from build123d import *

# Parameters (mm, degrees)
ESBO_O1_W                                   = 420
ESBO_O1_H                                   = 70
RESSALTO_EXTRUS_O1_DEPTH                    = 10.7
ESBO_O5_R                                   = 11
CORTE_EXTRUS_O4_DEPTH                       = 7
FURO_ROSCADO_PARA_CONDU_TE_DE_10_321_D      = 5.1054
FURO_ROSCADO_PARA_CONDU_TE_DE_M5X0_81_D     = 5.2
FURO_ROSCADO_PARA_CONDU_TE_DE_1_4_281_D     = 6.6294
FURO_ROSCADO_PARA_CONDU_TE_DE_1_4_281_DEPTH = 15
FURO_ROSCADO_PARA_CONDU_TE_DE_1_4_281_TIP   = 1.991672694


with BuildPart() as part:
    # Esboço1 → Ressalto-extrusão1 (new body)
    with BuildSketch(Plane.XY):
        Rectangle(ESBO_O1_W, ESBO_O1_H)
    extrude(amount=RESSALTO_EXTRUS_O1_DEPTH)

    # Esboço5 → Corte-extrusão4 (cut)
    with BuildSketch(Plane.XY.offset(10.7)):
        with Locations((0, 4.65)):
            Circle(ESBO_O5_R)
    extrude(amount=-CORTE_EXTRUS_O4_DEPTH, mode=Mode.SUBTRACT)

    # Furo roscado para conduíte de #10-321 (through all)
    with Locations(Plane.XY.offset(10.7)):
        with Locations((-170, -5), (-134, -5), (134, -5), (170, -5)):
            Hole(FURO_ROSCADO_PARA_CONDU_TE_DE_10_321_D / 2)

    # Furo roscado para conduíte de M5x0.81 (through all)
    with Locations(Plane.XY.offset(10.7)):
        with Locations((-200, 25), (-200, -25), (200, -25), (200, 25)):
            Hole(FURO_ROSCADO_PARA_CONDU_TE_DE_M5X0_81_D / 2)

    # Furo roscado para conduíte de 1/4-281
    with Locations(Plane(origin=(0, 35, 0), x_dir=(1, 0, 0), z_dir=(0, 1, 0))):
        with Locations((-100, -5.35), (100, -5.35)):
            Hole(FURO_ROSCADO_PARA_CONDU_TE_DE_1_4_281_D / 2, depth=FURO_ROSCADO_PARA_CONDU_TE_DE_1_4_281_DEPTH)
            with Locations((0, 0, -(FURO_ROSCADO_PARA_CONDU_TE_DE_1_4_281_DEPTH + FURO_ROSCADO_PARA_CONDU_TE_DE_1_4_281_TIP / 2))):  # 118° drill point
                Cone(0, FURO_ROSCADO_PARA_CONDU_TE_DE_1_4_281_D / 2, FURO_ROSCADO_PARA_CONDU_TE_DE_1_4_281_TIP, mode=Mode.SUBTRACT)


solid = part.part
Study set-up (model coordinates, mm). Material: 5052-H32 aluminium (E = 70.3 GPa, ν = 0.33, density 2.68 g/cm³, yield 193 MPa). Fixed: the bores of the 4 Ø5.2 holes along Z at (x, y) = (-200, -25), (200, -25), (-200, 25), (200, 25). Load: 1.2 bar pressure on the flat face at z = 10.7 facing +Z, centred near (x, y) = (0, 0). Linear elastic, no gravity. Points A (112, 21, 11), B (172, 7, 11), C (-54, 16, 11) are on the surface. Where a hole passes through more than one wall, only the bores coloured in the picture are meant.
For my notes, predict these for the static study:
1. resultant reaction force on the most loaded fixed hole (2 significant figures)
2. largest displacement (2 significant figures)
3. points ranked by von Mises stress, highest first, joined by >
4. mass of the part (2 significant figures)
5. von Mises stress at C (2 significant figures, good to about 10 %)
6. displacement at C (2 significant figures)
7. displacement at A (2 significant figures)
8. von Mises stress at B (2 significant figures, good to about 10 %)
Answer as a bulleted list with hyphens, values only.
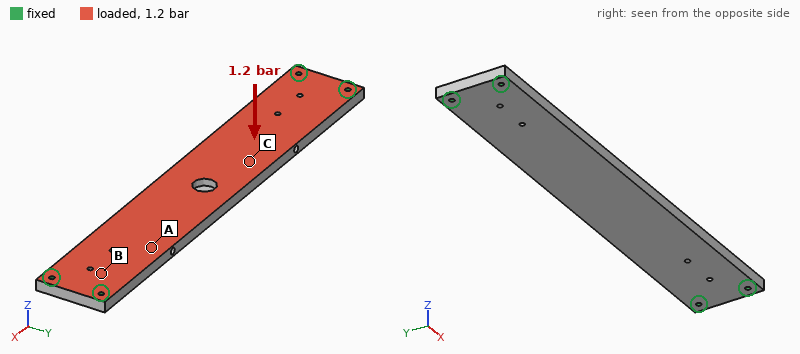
- 880 N
- 1.2 mm
- B > C > A
- 830 g
- 32 MPa
- 1.1 mm
- 0.59 mm
- 47 MPa
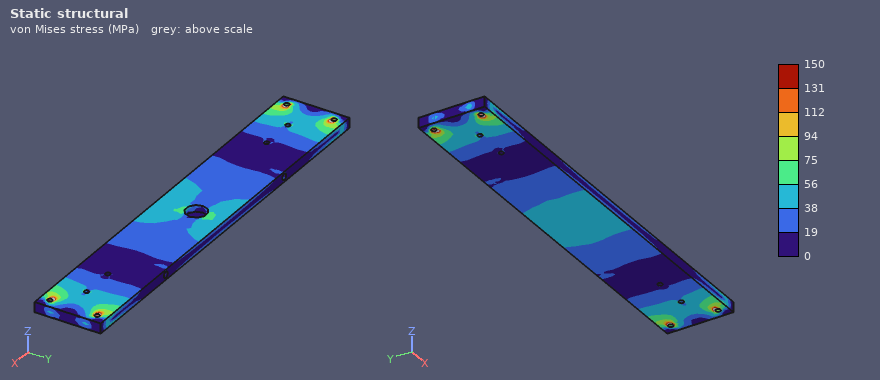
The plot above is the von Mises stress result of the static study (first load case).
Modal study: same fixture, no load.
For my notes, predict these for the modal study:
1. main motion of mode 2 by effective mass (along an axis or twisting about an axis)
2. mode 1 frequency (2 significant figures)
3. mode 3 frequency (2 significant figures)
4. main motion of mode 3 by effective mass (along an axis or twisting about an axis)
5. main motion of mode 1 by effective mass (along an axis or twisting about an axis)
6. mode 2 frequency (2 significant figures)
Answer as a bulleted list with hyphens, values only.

- twisting about Y
- 340 Hz
- 1200 Hz
- twisting about X
- along Z
- 930 Hz
